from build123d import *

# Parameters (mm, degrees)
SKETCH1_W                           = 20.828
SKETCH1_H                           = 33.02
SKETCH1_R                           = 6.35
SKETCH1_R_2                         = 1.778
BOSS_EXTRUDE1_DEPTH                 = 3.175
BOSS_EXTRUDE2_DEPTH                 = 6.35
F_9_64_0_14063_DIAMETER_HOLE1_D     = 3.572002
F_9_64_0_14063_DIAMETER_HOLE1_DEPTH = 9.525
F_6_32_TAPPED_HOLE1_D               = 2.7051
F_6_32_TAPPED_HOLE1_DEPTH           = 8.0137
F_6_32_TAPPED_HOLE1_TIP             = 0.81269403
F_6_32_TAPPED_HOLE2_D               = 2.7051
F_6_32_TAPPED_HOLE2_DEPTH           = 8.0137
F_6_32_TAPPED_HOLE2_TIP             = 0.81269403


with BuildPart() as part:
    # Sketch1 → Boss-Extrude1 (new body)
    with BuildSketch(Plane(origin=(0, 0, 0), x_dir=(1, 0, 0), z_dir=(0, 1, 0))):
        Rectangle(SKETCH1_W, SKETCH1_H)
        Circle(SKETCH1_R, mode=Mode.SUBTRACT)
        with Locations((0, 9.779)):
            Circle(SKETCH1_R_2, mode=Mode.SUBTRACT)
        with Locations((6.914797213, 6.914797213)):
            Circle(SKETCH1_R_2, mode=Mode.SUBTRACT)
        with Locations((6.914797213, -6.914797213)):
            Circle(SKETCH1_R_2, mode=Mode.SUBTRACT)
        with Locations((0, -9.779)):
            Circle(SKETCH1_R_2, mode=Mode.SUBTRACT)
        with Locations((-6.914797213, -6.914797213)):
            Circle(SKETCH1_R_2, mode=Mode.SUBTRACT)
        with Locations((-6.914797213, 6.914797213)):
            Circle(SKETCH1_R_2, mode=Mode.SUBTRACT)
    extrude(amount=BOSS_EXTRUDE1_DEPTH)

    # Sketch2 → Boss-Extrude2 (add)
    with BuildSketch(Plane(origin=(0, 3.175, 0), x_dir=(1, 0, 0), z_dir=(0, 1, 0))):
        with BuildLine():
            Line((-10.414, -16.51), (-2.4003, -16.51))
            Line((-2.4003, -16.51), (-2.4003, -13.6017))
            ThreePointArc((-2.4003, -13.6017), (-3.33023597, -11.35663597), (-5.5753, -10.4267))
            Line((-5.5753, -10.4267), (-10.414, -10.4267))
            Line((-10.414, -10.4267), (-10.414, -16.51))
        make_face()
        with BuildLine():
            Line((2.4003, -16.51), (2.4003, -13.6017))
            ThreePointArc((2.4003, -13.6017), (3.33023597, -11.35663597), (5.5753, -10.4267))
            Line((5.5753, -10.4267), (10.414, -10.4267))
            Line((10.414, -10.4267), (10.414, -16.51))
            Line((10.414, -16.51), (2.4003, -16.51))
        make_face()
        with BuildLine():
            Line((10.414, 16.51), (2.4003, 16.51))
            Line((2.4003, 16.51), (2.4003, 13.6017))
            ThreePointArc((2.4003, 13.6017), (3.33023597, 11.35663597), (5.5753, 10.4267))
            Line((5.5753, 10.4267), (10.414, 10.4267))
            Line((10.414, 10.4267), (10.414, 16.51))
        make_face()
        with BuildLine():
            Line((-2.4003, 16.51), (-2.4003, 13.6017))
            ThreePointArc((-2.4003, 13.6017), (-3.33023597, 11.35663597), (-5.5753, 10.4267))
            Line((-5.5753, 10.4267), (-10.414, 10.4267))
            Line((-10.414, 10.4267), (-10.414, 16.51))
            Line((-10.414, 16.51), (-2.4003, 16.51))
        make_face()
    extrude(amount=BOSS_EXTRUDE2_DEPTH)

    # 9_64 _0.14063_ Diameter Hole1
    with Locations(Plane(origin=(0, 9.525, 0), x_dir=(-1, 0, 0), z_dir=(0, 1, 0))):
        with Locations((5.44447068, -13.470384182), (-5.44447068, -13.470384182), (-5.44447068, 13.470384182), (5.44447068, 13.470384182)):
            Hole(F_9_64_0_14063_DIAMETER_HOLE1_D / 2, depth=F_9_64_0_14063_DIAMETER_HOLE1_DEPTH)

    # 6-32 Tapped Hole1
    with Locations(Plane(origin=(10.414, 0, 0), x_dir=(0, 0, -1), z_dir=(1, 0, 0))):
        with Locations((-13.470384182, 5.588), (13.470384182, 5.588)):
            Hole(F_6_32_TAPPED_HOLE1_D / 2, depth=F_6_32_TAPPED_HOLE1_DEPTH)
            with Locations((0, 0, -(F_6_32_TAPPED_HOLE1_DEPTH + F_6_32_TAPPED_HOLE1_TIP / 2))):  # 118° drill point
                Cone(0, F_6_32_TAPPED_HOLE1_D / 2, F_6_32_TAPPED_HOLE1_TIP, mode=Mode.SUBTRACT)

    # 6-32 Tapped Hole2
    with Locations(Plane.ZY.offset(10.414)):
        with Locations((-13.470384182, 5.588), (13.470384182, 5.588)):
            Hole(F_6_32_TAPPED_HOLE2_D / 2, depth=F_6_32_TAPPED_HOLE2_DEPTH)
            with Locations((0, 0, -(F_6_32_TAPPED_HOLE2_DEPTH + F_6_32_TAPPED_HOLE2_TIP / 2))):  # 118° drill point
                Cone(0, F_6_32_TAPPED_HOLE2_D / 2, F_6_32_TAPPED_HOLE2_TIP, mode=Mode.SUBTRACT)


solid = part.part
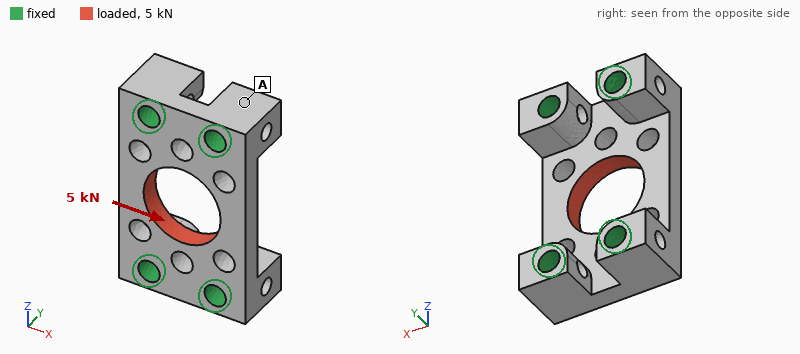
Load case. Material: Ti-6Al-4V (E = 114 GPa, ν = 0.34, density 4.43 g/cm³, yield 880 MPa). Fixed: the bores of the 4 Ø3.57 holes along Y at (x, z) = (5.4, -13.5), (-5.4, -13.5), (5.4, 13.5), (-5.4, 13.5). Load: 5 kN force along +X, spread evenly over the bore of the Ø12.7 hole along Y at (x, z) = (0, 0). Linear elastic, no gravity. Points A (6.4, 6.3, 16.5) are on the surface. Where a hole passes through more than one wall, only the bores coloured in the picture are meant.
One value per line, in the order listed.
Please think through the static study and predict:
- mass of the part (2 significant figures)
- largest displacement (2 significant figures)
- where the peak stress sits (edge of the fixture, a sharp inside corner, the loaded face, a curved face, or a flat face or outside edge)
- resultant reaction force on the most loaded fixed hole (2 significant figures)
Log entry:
10 g
24 µm
a curved face
1.3 kN
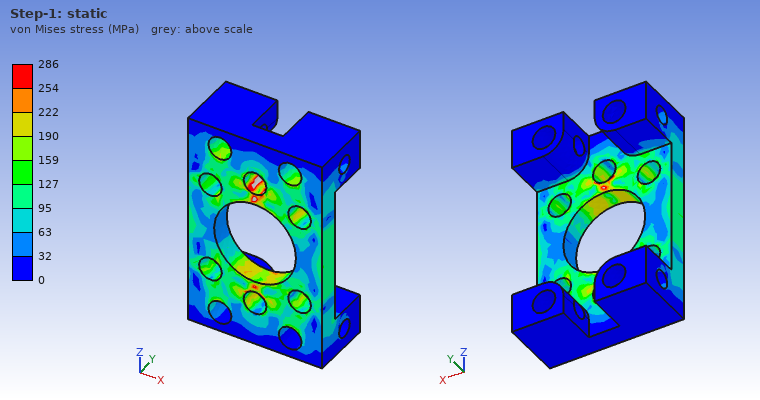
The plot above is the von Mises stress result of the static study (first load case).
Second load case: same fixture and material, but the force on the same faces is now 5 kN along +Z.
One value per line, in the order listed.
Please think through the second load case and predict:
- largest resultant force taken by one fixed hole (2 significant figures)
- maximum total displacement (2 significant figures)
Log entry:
1.3 kN
8.3 µm
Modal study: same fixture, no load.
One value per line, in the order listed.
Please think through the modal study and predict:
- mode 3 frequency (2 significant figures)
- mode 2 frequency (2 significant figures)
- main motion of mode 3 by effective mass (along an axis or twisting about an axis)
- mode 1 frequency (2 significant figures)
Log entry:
50 kHz
30 kHz
along X
29 kHz
